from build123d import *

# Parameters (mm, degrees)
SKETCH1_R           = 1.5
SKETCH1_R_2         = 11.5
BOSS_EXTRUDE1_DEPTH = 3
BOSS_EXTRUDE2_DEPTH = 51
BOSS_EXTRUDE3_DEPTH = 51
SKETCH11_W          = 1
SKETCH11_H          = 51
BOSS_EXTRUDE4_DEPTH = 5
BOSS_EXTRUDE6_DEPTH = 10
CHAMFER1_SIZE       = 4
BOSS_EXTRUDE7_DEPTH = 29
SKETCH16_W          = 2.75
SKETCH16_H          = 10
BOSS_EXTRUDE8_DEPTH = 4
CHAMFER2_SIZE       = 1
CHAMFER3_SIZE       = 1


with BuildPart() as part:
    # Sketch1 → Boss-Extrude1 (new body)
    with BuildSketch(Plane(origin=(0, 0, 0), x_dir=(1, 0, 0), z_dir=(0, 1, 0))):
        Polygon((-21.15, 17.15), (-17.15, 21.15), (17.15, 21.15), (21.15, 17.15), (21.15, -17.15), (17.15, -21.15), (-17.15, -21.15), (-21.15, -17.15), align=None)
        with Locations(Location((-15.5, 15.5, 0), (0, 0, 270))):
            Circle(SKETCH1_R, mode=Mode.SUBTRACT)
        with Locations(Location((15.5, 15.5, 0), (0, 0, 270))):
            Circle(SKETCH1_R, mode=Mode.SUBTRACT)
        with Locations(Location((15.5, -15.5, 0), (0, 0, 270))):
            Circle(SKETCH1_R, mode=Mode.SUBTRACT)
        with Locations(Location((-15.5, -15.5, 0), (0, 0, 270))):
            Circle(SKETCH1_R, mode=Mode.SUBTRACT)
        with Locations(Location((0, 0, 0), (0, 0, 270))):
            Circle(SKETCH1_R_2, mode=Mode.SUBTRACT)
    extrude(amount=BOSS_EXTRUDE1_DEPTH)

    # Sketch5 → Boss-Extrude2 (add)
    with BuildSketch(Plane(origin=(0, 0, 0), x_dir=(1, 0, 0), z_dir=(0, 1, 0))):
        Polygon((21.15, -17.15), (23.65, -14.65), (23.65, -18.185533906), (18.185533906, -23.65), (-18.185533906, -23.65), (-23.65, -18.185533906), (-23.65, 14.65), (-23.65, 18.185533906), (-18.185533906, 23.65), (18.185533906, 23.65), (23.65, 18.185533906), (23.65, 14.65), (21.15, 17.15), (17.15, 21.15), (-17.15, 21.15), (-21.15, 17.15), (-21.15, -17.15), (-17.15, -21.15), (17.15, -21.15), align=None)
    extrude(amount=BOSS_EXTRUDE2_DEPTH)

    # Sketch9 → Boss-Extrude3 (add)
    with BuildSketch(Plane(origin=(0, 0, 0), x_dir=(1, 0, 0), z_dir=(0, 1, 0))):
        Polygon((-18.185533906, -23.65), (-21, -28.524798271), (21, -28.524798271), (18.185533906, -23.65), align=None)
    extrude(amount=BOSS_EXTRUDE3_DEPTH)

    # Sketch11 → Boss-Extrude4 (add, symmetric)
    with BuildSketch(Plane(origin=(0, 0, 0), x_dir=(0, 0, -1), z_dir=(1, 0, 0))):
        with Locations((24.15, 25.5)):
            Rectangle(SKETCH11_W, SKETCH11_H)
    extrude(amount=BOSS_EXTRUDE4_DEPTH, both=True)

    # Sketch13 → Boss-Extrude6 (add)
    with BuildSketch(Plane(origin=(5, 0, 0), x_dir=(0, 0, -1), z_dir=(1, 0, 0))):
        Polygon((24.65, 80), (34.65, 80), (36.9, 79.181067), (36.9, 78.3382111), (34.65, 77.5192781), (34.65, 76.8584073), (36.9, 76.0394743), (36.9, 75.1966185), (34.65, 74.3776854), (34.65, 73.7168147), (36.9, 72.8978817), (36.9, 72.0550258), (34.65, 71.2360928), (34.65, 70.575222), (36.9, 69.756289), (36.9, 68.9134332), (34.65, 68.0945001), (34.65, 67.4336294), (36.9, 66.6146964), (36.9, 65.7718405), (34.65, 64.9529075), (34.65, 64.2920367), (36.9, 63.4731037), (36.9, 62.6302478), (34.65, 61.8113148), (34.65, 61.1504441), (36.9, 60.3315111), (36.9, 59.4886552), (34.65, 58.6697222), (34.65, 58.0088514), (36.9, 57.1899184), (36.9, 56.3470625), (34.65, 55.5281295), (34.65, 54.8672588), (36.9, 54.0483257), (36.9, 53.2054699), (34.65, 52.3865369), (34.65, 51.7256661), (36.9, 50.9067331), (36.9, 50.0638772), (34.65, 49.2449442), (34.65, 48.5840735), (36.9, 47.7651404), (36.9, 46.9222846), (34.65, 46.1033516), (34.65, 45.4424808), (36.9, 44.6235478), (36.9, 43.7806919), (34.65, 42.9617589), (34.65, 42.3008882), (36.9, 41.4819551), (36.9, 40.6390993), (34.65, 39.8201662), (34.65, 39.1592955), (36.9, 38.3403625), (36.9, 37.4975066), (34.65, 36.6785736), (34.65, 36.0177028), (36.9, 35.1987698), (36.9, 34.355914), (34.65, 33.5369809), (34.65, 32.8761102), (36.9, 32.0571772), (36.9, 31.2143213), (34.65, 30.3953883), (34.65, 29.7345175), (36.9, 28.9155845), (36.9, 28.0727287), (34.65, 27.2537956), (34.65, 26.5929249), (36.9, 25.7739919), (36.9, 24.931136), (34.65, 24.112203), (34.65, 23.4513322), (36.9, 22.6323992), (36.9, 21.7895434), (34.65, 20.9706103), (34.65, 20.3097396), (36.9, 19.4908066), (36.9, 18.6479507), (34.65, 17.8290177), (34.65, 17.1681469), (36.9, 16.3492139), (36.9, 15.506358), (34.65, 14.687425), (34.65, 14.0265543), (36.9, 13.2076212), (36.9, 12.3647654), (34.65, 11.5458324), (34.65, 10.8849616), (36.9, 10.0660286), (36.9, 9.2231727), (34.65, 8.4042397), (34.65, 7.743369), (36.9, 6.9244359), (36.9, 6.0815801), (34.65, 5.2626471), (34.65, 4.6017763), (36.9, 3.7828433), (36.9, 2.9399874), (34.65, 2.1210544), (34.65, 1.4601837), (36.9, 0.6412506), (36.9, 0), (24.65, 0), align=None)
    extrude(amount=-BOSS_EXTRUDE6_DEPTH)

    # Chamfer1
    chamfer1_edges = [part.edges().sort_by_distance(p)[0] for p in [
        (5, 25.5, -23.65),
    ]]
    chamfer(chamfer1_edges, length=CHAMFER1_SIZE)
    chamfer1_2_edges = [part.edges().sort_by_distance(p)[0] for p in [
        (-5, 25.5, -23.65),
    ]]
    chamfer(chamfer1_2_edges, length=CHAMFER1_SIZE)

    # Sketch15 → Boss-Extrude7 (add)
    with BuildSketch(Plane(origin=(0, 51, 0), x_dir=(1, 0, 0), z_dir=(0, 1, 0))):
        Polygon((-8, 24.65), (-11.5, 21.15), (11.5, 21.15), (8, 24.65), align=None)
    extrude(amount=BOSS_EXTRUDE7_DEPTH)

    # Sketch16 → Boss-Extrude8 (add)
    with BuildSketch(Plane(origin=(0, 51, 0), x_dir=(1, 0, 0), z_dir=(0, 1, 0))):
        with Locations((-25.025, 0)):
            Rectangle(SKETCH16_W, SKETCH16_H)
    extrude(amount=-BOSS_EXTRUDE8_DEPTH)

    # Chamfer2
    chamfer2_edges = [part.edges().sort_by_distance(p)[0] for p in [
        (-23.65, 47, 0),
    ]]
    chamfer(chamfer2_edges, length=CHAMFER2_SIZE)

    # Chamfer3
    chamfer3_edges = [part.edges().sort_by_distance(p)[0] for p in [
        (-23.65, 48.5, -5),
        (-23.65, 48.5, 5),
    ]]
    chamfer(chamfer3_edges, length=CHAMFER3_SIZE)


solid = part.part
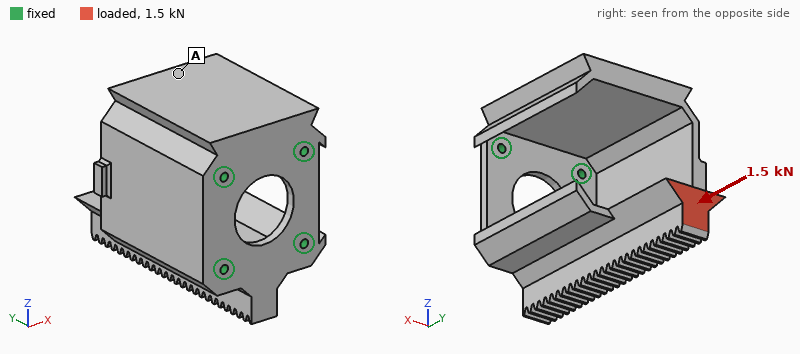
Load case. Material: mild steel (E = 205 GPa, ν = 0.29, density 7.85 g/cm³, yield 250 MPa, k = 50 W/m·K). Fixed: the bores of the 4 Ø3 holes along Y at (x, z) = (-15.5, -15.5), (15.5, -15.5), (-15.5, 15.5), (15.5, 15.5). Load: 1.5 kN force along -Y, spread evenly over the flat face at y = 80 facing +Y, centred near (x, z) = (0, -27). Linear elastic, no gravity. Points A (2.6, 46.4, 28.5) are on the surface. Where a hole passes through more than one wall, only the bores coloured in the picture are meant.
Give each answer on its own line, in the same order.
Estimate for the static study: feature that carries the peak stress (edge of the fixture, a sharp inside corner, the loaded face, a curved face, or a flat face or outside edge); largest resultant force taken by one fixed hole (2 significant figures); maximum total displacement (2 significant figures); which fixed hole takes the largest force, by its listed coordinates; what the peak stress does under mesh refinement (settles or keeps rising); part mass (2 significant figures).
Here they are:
edge of the fixture
1.2 kN
79 µm
(-15.5, -15.5)
keeps rising
340 g
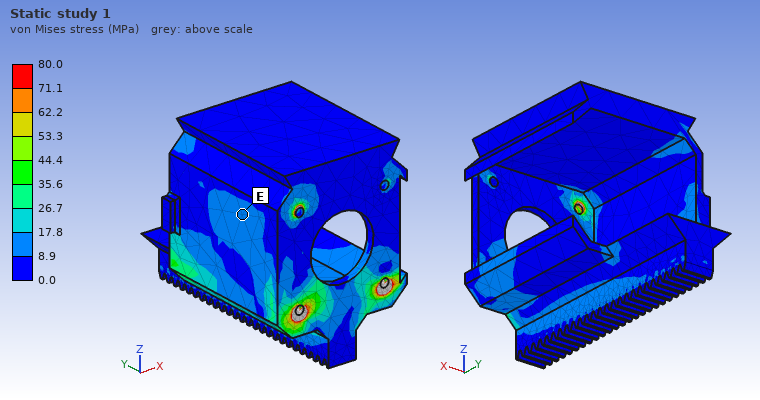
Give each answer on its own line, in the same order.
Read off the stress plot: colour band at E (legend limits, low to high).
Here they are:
8.9 to 17.8 MPa
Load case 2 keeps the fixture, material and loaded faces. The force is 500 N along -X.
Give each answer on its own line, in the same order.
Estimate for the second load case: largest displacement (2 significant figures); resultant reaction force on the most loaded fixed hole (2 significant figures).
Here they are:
61 µm
1.2 kN
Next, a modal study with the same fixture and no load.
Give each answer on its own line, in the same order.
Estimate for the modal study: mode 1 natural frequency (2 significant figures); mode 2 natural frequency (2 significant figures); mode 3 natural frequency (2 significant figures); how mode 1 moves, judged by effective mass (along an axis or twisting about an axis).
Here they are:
1100 Hz
2000 Hz
2700 Hz
along Z
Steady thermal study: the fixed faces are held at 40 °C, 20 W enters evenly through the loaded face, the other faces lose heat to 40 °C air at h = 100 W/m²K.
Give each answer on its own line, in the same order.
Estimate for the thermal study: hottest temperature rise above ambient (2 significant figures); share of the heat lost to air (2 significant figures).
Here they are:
71 K
90 %
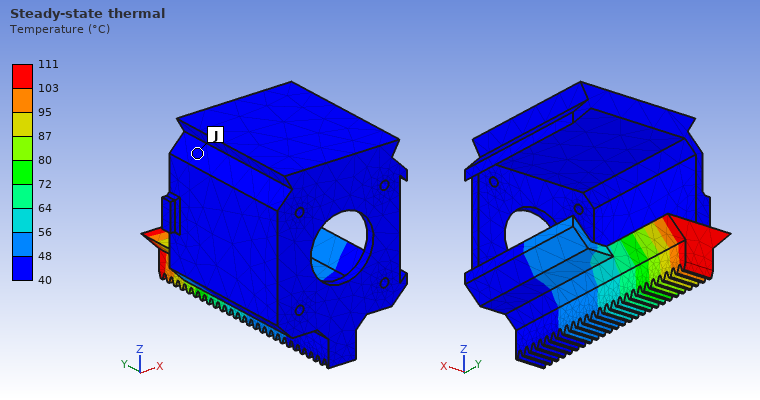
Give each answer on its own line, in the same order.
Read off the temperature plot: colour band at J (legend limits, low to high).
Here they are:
40 to 48 °C
